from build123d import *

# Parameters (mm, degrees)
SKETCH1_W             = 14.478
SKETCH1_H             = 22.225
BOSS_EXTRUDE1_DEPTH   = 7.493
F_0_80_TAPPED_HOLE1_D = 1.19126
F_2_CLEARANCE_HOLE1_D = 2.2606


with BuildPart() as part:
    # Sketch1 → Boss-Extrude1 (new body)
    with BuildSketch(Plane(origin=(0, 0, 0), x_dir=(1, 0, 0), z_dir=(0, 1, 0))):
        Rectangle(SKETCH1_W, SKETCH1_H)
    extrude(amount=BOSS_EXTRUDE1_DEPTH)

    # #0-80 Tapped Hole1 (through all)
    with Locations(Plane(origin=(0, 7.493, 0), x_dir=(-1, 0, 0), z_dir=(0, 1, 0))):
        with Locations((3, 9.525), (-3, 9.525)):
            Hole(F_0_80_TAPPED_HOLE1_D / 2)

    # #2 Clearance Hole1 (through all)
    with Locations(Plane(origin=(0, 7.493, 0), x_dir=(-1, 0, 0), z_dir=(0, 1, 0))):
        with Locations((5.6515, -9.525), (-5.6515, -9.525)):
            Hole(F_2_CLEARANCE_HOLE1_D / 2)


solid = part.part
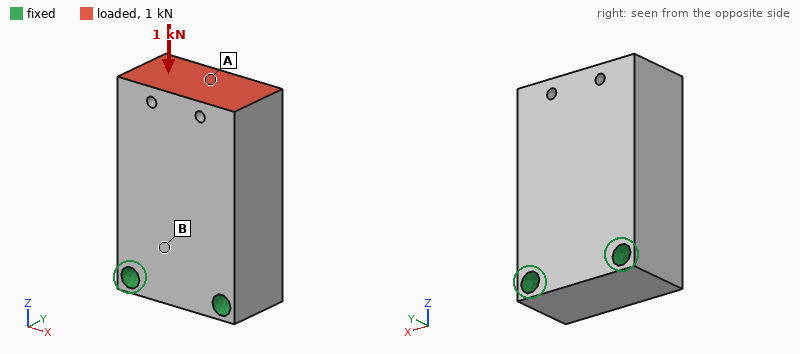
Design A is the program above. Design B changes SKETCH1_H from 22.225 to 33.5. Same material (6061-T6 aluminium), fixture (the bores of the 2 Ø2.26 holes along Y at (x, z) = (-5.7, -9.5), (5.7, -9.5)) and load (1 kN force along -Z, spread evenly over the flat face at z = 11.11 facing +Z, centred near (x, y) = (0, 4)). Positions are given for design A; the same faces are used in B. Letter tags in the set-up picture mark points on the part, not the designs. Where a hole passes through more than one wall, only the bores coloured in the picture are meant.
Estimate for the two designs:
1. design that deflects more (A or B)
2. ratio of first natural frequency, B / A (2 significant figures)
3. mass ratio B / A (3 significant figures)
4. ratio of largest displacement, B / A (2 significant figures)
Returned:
B
0.66
1.52
1.2
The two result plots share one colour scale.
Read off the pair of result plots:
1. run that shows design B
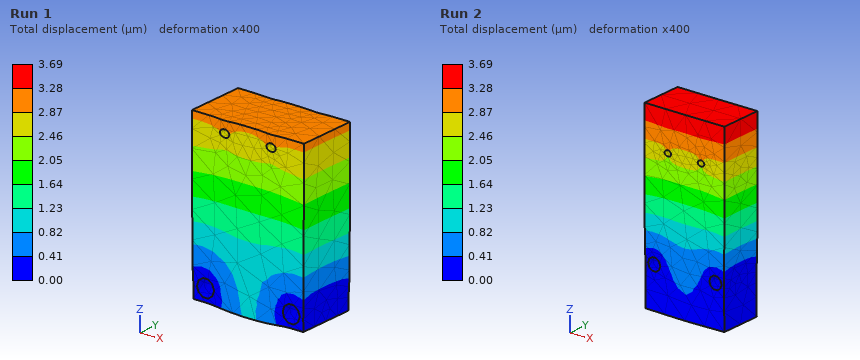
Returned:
Run 2
